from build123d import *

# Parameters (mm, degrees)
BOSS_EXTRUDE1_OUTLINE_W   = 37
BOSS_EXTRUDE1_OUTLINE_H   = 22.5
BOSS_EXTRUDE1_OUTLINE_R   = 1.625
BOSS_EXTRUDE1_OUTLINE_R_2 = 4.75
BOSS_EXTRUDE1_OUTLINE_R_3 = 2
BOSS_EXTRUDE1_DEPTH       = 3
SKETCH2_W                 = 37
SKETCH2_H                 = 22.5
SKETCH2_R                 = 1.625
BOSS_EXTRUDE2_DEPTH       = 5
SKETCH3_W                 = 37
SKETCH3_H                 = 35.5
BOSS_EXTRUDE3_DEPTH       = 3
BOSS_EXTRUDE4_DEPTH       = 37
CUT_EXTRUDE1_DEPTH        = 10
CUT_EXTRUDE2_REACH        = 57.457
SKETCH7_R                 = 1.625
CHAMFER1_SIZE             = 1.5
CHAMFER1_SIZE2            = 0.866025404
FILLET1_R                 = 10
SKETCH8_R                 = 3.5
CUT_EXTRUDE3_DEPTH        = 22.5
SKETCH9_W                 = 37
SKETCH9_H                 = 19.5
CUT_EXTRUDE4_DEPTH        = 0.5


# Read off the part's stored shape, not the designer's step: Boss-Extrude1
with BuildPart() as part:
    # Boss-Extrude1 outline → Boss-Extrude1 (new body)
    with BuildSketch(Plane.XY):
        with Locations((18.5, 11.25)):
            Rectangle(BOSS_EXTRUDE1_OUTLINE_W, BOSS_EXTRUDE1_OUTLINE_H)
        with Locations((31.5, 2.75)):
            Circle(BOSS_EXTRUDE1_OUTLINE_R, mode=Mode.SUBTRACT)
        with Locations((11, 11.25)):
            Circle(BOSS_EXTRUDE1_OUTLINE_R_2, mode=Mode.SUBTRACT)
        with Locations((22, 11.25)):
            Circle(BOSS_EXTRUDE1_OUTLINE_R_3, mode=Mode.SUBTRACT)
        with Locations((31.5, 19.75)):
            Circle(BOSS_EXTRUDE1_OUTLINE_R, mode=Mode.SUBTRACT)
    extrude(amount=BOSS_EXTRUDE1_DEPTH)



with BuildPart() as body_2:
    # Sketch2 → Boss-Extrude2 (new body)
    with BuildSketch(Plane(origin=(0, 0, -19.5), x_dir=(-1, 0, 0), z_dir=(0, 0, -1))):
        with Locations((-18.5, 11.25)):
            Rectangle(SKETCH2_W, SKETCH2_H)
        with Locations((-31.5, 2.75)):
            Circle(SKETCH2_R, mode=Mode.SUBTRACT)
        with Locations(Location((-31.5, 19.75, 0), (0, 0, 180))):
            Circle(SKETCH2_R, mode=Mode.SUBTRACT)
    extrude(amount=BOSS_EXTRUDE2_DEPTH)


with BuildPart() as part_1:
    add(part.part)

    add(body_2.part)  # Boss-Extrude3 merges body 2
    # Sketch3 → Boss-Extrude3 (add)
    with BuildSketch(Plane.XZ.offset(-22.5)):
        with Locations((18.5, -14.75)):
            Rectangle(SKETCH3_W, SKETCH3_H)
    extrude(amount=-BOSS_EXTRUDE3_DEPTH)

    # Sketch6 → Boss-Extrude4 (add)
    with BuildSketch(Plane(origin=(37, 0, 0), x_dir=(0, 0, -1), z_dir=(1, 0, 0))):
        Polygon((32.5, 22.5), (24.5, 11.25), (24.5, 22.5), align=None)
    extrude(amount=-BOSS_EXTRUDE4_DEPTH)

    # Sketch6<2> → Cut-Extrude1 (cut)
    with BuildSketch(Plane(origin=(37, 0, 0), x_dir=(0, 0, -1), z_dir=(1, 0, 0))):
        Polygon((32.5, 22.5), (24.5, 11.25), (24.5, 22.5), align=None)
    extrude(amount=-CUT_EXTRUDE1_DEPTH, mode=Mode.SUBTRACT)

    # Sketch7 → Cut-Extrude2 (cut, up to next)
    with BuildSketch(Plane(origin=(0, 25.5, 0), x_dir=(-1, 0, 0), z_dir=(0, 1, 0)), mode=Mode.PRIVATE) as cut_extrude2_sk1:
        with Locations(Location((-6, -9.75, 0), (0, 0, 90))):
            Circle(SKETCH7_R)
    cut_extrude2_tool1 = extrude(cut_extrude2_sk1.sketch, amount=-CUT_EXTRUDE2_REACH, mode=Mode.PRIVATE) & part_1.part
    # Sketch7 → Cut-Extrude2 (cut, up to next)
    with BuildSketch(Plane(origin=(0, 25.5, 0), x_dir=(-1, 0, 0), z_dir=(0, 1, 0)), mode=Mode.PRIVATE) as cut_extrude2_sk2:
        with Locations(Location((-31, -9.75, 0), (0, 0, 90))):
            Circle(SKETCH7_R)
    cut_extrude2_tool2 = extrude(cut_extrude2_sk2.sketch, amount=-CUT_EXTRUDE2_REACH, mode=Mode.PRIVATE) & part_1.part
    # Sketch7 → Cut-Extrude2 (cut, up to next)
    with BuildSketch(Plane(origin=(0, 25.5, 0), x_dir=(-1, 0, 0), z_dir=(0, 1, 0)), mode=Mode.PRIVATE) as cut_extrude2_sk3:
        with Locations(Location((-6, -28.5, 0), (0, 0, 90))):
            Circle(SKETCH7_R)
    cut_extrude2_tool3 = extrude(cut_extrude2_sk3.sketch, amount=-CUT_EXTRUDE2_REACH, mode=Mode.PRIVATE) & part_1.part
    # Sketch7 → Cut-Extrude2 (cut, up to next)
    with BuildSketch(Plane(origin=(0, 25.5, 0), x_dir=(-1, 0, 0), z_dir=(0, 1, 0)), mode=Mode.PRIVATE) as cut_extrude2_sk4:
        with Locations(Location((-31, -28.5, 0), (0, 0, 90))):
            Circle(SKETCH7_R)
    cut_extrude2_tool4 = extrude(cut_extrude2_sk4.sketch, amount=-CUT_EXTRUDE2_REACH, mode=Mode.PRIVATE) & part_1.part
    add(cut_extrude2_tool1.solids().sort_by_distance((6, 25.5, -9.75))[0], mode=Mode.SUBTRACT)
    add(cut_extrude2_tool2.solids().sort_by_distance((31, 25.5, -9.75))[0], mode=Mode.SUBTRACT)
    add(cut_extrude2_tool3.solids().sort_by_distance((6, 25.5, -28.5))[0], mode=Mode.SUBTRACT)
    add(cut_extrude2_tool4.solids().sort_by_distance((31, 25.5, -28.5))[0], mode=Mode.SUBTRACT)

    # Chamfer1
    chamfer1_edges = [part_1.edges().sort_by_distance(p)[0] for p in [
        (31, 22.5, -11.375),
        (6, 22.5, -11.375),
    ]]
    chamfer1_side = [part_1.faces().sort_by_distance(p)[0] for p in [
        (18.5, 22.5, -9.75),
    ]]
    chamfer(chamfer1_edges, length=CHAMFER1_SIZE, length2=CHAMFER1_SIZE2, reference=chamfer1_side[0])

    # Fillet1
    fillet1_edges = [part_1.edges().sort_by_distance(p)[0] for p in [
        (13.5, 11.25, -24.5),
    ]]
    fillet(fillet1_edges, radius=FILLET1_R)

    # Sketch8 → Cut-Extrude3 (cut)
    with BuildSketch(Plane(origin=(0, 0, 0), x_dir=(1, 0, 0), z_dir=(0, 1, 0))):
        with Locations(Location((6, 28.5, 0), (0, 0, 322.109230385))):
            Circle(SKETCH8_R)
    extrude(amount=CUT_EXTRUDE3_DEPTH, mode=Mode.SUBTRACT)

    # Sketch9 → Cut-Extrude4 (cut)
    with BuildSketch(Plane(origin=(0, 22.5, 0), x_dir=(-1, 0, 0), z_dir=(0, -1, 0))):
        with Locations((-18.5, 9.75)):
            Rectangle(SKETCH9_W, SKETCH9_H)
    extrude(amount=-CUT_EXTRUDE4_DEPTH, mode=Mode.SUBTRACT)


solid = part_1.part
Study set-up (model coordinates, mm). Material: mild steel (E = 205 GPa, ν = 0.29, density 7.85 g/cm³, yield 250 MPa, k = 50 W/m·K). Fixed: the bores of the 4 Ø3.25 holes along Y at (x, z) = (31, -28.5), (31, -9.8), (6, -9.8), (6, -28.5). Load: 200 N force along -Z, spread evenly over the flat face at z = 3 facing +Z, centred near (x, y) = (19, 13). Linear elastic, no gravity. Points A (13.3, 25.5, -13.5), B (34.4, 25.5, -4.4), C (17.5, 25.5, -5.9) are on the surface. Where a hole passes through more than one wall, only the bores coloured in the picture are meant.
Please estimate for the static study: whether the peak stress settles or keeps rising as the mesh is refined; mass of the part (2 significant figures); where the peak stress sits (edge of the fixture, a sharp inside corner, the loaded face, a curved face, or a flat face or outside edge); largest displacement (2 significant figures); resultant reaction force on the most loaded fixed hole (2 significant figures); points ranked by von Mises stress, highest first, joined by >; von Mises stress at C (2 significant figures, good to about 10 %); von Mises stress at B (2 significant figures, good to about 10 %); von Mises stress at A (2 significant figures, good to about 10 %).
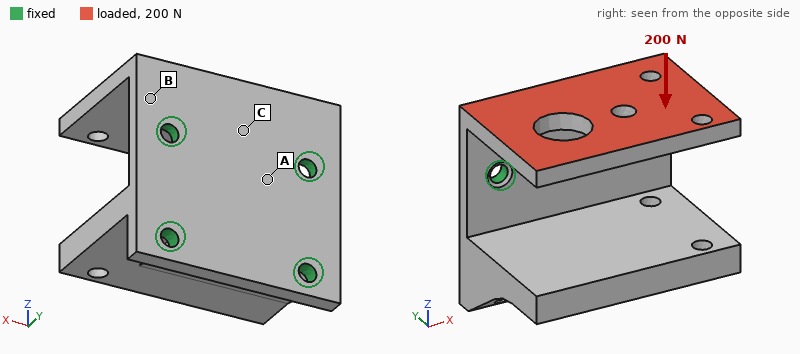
keeps rising
85 g
edge of the fixture
82 µm
80 N
B > C > A
41 MPa
58 MPa
11 MPa
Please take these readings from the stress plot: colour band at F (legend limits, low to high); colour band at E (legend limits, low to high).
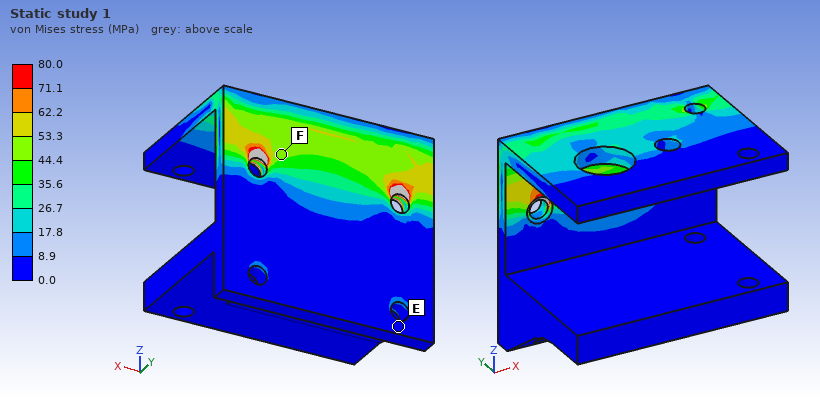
44.4 to 53.3 MPa
0.0 to 8.9 MPa
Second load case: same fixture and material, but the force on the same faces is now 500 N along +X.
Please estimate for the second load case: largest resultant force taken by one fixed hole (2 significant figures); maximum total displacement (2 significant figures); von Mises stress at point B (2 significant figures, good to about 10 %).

400 N
28 µm
31 MPa
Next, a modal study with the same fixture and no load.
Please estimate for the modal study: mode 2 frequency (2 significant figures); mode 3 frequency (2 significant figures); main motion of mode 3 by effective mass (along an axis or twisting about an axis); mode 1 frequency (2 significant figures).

4500 Hz
6600 Hz
along Z
2100 Hz
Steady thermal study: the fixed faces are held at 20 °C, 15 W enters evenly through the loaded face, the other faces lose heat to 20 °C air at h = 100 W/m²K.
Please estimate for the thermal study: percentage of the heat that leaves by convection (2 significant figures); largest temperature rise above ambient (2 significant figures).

43 %
47 K
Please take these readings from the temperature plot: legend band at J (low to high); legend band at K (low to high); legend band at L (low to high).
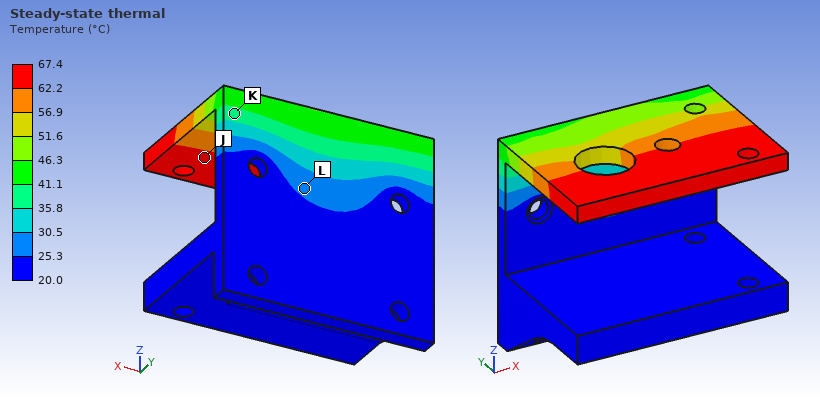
62.2 to 67.4 °C
35.8 to 41.1 °C
25.3 to 30.5 °C
